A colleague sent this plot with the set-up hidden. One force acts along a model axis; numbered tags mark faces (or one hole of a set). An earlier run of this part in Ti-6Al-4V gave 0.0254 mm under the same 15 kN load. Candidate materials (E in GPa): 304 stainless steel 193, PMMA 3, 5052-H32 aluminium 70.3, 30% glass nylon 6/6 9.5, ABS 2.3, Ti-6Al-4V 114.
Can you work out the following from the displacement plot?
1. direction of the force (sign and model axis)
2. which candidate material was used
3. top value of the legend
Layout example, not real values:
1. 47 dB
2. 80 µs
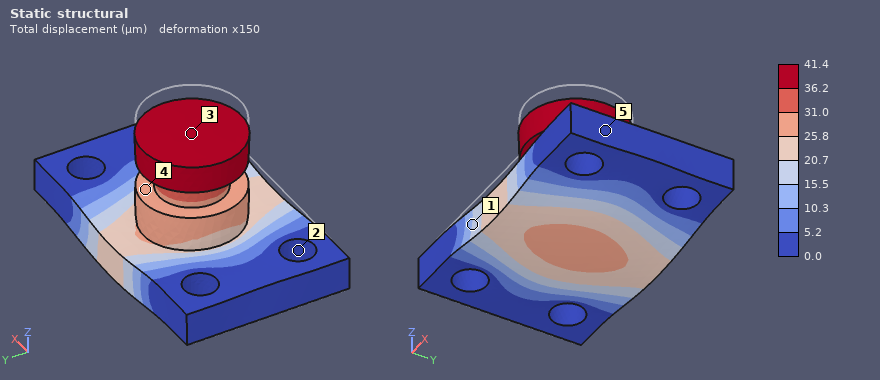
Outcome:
1. -Z
2. 5052-H32 aluminium
3. 41.4 µm
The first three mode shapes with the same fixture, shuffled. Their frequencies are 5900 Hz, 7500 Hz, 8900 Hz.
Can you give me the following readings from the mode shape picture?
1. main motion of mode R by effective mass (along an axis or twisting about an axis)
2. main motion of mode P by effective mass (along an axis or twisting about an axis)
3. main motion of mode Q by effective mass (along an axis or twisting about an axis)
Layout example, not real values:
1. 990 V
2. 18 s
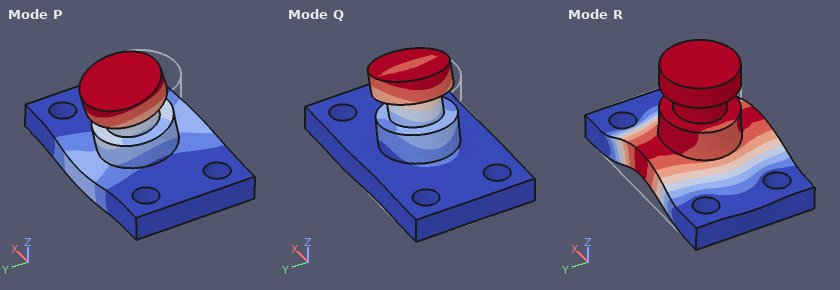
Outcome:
1. along Z
2. along Y
3. along X
